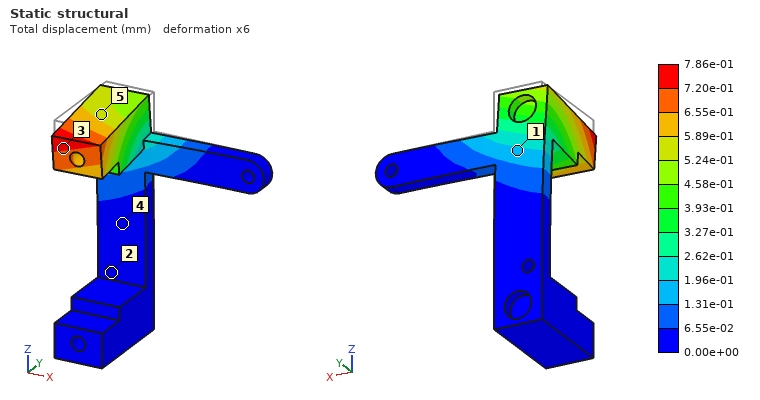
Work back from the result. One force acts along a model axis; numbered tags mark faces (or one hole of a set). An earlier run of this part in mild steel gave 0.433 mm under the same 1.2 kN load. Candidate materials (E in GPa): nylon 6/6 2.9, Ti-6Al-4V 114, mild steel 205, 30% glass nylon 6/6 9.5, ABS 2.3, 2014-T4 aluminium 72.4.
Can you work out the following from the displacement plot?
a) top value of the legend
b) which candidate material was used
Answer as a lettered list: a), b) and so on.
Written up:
a) 7.86e-01 mm
b) Ti-6Al-4V
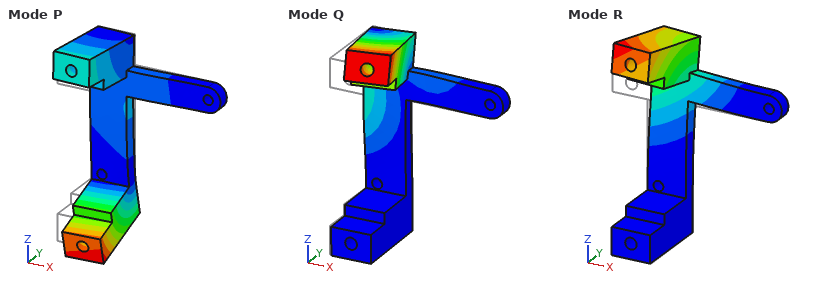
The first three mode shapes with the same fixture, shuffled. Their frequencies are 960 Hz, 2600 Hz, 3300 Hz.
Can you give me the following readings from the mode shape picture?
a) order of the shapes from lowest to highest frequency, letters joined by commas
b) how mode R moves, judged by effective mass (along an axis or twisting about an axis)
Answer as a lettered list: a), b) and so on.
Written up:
a) R, Q, P
b) along Y
